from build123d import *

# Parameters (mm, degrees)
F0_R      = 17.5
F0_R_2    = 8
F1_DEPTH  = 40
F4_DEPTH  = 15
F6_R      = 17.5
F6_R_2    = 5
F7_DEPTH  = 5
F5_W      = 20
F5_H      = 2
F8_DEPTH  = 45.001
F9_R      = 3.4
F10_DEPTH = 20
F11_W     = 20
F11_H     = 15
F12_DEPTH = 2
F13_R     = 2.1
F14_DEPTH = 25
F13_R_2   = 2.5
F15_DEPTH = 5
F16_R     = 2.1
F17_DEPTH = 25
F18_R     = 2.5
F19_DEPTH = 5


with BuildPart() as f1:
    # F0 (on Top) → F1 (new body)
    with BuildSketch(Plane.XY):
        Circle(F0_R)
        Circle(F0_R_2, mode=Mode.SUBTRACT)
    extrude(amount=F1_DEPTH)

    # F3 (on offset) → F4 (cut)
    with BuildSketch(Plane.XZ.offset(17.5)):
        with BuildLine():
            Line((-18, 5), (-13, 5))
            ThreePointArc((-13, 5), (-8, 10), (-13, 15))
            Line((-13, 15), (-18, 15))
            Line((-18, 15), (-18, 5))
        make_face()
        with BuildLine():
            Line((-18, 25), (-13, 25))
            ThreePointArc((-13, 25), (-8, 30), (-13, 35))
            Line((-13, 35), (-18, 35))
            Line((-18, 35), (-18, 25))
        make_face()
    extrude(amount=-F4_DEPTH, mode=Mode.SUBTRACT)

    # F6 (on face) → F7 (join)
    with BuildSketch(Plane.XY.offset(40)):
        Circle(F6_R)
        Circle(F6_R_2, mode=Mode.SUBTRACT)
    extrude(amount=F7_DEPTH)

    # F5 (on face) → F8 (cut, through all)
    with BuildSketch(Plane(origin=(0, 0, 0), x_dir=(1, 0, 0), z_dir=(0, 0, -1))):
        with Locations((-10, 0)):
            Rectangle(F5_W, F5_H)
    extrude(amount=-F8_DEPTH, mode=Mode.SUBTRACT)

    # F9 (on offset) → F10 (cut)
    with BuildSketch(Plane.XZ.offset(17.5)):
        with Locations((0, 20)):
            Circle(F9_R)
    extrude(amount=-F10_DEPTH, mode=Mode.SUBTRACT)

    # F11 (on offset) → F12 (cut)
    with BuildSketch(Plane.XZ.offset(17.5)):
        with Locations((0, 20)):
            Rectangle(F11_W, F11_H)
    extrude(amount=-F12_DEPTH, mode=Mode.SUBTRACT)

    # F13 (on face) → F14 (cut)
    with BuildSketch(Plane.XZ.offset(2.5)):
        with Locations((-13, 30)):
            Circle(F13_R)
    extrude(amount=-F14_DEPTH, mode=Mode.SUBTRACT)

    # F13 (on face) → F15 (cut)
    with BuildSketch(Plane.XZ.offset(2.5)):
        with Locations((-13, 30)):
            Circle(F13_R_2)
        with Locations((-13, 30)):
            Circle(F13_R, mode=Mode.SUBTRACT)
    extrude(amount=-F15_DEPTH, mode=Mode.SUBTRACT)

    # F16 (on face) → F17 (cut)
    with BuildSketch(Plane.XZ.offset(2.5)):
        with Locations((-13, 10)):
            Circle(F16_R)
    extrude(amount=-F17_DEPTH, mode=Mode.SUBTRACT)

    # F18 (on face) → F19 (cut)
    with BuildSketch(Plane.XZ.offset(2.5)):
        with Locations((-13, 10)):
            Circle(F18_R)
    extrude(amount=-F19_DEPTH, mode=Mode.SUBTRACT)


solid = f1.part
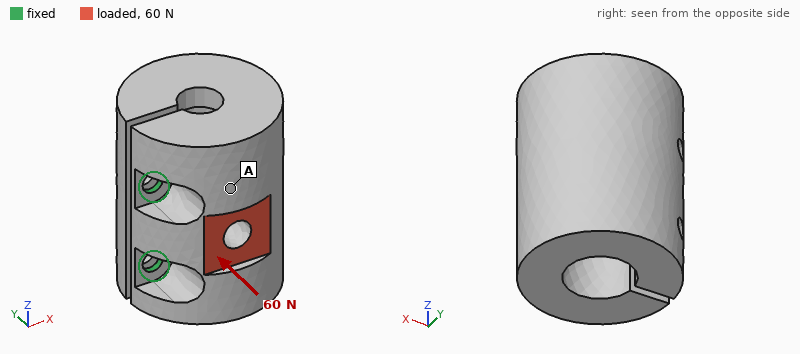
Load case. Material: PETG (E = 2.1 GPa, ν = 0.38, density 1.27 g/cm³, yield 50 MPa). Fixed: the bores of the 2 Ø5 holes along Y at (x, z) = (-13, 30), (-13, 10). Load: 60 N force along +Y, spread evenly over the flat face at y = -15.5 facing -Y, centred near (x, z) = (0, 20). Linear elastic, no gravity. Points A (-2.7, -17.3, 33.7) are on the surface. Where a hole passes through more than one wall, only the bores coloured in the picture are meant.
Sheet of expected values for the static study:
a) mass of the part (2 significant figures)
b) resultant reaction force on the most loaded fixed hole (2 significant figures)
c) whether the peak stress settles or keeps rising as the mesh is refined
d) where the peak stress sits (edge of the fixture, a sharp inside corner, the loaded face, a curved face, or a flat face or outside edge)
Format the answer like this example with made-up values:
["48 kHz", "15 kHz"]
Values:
["40 g", "30 N", "keeps rising", "edge of the fixture"]
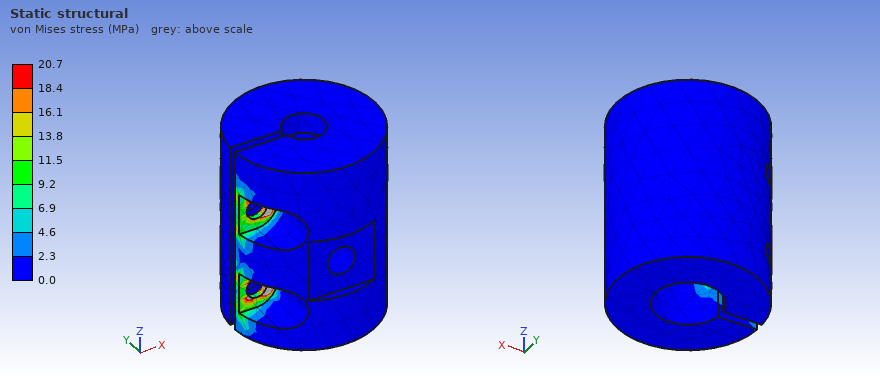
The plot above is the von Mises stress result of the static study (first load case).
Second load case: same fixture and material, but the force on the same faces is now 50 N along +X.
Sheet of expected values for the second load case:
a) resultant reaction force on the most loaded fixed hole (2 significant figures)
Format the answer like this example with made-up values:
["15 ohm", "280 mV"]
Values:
["25 N"]
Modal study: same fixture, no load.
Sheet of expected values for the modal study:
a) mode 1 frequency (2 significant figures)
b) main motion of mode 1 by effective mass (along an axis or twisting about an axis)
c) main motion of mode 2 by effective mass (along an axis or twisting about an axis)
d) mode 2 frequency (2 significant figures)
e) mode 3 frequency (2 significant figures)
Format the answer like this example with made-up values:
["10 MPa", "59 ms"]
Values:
["240 Hz", "along Y", "along Z", "540 Hz", "790 Hz"]
